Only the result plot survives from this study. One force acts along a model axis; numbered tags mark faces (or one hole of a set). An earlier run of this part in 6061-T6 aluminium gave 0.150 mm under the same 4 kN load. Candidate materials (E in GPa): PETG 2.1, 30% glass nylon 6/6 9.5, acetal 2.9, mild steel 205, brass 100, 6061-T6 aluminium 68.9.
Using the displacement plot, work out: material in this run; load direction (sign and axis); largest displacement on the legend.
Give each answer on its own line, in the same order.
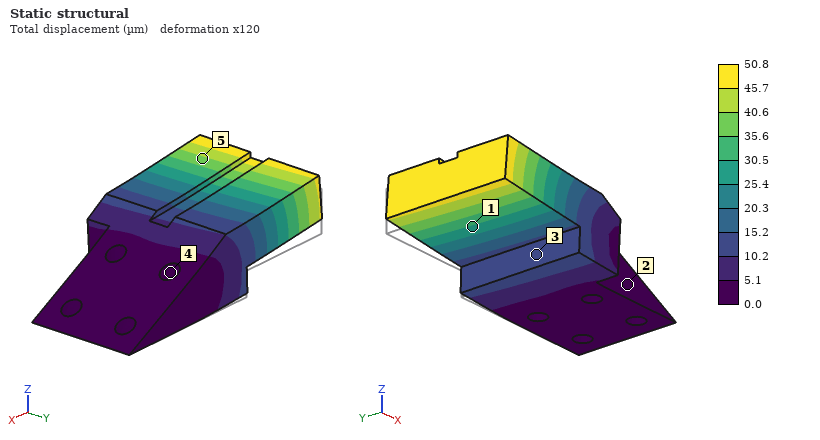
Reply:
mild steel
+Z
50.8 µm
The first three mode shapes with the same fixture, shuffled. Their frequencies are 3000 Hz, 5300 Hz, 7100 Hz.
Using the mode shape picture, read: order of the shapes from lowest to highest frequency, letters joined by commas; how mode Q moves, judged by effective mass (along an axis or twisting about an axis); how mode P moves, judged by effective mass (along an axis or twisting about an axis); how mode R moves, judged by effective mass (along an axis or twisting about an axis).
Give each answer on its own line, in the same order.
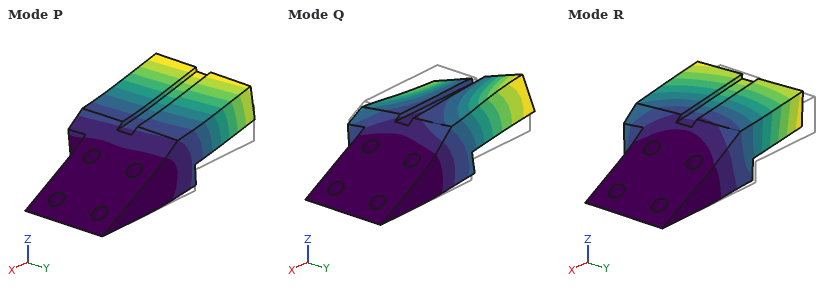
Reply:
P, R, Q
twisting about X
along Z
along Y
